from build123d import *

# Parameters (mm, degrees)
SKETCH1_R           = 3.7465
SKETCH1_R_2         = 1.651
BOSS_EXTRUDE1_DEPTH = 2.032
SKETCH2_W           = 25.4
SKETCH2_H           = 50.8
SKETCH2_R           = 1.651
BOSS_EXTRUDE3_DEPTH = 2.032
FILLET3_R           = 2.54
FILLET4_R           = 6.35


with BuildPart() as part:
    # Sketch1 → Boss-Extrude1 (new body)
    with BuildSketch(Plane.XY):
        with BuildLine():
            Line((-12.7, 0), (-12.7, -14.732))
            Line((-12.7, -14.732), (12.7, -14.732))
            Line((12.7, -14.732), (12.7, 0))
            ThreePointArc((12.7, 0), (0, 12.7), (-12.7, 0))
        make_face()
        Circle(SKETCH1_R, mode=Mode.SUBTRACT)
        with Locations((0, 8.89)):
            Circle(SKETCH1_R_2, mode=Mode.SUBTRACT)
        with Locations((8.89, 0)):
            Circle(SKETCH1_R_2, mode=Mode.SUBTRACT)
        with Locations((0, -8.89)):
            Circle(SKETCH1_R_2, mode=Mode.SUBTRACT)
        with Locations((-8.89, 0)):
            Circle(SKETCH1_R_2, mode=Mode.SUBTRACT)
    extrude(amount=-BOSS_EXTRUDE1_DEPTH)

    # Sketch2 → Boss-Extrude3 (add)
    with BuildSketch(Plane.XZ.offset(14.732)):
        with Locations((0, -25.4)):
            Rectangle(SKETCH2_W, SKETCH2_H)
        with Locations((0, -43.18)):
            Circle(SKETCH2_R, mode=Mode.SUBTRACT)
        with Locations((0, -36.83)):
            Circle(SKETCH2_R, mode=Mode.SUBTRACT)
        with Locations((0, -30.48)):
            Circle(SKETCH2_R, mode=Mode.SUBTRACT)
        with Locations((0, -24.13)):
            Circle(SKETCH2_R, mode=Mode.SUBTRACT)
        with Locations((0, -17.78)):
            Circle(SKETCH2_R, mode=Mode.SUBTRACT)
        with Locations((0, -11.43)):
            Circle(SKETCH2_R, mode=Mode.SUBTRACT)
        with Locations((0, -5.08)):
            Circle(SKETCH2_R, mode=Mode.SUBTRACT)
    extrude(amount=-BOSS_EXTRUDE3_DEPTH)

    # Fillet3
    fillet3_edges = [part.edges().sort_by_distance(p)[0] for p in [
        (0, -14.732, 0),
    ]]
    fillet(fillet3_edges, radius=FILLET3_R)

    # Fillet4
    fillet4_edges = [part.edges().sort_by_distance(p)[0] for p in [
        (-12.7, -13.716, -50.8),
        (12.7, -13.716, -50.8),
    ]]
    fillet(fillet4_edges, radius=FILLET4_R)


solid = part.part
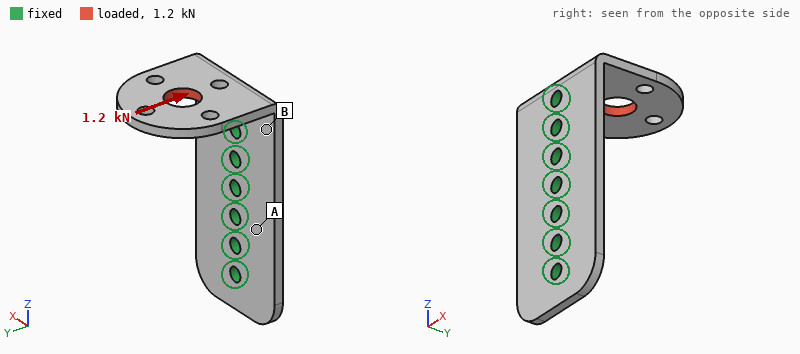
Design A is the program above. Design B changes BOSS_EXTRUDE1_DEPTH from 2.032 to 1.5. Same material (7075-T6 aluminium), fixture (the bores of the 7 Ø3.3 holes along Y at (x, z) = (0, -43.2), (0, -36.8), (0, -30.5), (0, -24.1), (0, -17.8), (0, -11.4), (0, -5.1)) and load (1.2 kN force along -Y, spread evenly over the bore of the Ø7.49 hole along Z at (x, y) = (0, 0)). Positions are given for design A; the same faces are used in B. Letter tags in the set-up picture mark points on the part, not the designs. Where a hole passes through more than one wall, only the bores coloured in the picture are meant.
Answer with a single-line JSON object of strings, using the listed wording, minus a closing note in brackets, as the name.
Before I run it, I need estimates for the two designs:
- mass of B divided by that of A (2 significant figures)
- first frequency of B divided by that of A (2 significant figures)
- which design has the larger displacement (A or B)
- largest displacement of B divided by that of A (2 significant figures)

{"mass of B divided by that of A": "0.92", "first frequency of B divided by that of A": "0.83", "which design has the larger displacement": "B", "largest displacement of B divided by that of A": "1.2"}
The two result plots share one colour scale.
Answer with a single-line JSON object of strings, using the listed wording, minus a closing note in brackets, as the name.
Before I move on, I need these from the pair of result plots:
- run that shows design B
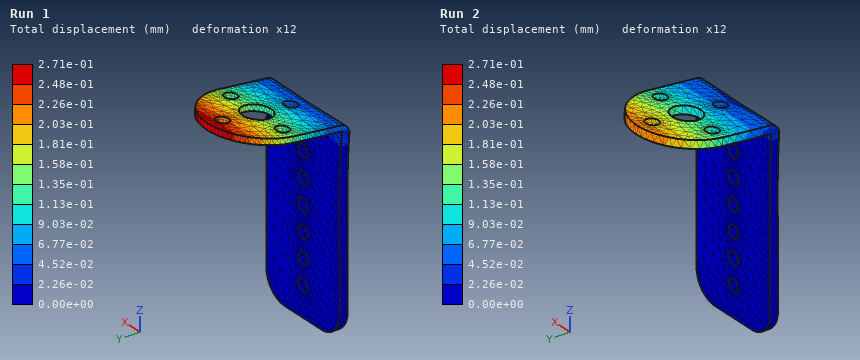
{"run that shows design B": "Run 1"}
